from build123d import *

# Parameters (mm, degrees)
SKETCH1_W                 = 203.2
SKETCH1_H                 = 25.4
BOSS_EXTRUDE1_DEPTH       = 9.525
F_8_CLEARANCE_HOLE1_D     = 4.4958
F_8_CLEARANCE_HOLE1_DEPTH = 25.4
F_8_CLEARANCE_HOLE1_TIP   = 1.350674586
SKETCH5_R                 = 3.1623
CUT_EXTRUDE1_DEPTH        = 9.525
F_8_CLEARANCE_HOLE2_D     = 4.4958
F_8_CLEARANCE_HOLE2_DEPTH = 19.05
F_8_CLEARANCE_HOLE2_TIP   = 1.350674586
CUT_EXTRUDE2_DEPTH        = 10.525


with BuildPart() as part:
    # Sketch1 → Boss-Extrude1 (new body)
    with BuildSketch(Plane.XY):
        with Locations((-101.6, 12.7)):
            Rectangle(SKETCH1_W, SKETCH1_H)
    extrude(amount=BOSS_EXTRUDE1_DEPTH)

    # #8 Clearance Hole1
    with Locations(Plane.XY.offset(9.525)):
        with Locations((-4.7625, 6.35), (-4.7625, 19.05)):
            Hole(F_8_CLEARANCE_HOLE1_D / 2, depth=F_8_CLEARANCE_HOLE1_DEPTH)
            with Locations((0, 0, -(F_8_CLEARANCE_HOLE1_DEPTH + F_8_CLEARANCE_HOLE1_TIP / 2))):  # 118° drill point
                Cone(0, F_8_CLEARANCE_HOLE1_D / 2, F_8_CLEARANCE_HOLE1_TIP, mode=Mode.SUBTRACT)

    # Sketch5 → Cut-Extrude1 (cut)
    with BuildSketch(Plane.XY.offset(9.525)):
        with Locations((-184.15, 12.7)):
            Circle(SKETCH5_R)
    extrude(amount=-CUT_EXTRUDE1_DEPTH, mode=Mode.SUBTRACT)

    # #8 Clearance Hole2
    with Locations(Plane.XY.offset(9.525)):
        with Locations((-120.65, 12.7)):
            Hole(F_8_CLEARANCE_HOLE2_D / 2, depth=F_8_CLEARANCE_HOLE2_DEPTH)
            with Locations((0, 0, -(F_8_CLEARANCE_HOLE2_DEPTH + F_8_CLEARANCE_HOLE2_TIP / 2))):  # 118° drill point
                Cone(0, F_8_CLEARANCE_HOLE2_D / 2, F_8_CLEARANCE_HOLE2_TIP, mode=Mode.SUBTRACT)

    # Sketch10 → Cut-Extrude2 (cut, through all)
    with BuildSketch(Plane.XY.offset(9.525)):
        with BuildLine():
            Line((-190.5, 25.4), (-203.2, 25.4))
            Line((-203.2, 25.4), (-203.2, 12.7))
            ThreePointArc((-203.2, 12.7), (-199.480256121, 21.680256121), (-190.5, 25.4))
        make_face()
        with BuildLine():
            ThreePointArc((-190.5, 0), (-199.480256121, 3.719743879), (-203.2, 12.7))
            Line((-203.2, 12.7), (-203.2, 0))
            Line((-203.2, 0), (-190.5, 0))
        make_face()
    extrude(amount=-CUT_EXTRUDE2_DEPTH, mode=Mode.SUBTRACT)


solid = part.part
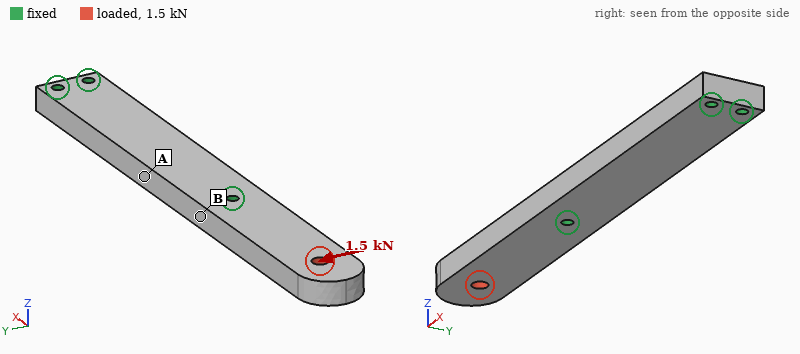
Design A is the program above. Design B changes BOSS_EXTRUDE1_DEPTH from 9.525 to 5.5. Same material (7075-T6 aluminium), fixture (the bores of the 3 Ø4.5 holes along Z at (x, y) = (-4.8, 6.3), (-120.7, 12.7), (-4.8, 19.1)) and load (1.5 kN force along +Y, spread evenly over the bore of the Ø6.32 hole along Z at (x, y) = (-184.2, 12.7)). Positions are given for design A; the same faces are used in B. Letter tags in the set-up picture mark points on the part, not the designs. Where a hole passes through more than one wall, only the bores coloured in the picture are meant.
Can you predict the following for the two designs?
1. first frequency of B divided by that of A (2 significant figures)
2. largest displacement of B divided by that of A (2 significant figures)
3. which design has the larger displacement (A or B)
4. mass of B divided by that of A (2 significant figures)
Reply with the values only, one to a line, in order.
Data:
0.60
1.7
B
0.58
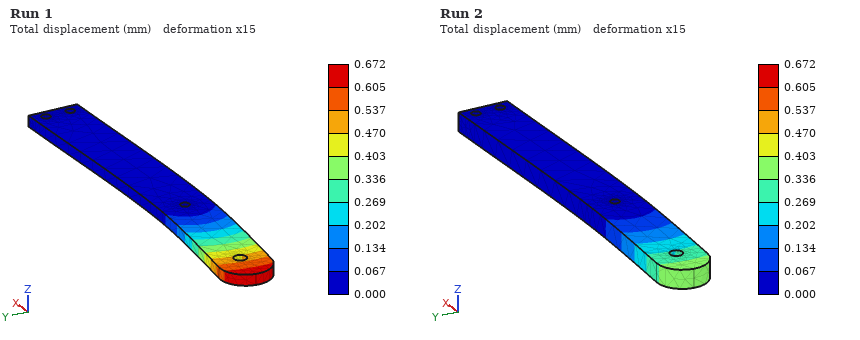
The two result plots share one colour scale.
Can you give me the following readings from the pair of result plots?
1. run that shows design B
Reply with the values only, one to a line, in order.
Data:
Run 1
